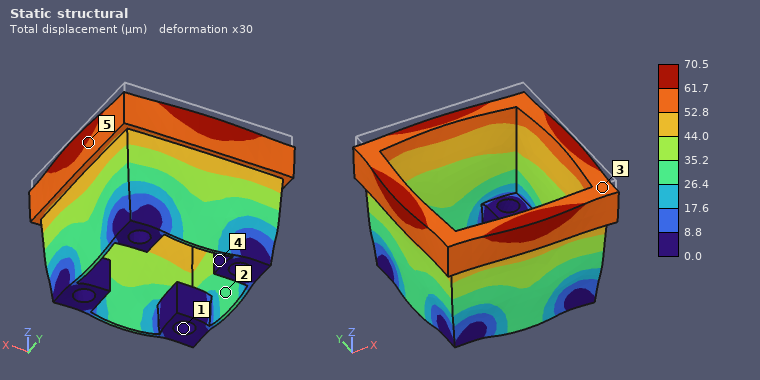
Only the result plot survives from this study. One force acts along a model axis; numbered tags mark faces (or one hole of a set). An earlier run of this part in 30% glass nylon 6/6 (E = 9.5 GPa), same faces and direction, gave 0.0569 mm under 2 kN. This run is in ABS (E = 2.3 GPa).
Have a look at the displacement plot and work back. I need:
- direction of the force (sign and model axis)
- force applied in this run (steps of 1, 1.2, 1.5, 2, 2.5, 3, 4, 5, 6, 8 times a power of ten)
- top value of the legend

-Z
600 N
70.5 µm
